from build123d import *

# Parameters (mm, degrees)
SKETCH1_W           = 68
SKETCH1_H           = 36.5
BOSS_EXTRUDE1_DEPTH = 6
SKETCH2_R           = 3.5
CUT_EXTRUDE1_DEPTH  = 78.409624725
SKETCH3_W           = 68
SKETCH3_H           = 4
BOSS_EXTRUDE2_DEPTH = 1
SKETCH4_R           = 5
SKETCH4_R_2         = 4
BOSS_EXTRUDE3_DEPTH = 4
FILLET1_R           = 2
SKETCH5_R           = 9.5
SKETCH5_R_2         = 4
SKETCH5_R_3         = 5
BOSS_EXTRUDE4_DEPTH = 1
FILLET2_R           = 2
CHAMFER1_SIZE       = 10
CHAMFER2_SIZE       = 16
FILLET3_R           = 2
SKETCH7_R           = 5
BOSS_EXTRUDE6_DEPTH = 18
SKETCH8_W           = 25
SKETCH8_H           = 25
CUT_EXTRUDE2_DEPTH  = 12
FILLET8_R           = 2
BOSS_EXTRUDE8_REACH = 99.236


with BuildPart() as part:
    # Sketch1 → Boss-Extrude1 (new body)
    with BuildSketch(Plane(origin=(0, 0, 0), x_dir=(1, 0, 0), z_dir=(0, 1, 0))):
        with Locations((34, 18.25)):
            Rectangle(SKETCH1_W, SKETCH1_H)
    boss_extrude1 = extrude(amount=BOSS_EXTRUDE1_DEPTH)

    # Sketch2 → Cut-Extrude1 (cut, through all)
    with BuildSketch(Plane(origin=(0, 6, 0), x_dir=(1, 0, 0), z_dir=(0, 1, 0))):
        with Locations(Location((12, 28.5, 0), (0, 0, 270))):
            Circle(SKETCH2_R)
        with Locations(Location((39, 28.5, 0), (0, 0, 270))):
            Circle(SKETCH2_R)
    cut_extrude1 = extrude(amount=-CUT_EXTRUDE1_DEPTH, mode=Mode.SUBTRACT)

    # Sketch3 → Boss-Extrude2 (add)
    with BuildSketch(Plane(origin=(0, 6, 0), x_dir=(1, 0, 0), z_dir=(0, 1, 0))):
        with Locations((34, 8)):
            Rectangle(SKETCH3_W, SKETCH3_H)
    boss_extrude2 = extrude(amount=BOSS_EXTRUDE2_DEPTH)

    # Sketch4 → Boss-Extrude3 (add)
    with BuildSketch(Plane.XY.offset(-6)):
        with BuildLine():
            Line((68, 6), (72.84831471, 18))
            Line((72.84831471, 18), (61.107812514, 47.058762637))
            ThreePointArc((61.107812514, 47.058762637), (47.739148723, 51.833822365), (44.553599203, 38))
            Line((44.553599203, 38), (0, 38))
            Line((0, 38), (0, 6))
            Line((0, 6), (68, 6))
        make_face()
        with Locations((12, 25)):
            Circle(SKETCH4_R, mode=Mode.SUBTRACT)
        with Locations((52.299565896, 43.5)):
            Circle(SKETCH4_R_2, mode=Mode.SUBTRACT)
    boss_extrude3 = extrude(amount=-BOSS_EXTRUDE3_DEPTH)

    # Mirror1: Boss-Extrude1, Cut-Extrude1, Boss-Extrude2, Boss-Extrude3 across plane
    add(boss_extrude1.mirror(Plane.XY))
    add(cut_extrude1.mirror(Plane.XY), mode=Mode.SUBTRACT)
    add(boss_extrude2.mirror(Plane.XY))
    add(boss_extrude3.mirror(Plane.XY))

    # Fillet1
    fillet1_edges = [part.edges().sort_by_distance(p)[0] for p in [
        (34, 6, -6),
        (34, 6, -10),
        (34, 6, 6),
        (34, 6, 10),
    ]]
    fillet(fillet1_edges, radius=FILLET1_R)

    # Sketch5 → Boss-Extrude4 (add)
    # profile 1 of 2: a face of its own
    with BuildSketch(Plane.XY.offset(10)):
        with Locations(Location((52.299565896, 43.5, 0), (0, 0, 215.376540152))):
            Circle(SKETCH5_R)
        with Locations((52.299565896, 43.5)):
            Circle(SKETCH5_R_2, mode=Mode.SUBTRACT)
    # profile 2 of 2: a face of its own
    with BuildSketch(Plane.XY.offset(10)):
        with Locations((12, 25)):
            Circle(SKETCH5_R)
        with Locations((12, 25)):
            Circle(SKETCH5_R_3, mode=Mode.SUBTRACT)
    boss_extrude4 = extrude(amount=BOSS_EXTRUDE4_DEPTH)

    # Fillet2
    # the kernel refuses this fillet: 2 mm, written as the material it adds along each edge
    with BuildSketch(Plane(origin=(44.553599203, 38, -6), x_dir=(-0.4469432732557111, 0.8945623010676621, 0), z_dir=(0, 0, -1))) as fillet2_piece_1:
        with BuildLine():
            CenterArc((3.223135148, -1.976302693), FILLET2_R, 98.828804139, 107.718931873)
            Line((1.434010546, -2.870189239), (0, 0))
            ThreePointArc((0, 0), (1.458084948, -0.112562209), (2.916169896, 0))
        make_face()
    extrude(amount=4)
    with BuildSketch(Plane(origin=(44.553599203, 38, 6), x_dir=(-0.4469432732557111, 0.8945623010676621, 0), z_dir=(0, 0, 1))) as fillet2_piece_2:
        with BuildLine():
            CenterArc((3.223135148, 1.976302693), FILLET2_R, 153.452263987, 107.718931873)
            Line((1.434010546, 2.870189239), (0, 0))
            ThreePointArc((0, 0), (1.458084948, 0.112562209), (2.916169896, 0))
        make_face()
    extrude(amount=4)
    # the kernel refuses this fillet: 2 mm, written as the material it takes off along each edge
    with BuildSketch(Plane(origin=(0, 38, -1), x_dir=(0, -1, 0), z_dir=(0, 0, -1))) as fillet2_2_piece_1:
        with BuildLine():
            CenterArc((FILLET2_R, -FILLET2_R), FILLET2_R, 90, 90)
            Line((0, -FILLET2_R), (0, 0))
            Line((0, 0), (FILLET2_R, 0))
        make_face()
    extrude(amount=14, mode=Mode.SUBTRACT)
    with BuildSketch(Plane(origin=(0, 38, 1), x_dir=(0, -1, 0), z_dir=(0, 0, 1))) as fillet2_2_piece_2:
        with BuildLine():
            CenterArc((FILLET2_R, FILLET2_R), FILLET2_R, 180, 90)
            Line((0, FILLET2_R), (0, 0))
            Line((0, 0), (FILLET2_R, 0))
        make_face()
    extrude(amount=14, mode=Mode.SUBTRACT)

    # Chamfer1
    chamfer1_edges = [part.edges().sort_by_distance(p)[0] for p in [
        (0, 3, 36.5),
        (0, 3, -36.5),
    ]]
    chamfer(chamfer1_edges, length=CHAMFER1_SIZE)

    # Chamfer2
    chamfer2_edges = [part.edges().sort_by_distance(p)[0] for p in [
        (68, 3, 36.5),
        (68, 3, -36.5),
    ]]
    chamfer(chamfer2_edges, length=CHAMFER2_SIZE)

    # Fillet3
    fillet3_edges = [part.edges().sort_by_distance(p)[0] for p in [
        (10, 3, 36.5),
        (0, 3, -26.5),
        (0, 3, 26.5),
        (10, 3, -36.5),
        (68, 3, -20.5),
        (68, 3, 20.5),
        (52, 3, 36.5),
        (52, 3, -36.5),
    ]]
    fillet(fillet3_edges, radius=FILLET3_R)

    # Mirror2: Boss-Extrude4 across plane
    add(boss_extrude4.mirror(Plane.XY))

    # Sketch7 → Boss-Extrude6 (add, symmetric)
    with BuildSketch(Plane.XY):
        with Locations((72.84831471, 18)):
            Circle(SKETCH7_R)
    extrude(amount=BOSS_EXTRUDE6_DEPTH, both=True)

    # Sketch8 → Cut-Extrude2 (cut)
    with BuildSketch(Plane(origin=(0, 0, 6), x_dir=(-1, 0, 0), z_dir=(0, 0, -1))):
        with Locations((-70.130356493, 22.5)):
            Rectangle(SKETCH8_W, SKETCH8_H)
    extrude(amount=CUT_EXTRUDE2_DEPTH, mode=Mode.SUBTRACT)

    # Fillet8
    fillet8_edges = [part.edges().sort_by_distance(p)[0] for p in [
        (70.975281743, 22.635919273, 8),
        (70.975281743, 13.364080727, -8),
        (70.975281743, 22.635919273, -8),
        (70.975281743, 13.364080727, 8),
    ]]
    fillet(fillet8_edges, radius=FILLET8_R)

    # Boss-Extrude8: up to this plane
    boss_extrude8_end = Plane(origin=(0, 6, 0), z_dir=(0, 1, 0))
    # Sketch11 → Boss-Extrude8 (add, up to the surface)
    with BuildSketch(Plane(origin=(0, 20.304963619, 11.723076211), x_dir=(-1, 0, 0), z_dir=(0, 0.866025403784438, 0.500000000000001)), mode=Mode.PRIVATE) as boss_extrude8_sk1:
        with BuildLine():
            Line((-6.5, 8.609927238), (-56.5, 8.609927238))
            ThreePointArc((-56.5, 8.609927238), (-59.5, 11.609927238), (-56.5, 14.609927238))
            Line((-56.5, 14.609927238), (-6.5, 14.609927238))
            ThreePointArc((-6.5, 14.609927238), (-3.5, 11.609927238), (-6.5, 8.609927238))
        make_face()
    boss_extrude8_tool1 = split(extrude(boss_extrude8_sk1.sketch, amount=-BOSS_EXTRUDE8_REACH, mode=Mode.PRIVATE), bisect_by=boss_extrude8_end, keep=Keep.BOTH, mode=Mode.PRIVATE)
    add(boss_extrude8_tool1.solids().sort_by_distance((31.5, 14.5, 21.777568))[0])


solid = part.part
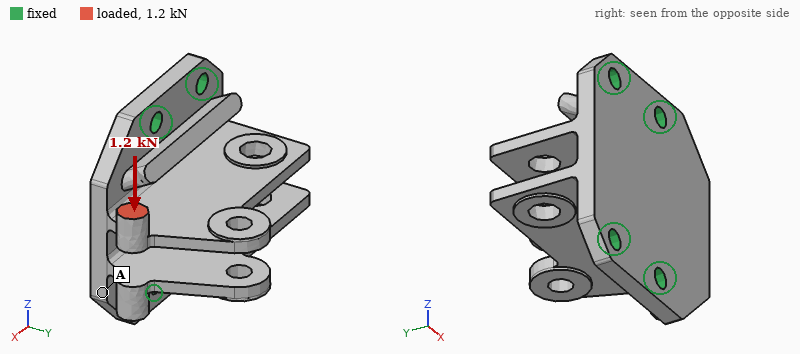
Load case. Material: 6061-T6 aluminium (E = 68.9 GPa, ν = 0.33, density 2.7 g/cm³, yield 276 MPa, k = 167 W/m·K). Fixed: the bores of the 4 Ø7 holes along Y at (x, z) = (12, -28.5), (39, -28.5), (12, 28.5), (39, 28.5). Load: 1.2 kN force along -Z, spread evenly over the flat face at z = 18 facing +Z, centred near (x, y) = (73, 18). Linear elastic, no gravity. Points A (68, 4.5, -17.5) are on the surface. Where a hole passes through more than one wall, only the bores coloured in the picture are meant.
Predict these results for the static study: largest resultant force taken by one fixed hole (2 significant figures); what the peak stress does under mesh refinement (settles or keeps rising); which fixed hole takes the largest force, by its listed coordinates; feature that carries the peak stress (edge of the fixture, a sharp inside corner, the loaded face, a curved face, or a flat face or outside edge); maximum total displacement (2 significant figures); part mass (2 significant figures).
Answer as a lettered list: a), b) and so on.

a) 1.1 kN
b) keeps rising
c) (39, 28.5)
d) a sharp inside corner
e) 0.43 mm
f) 140 g
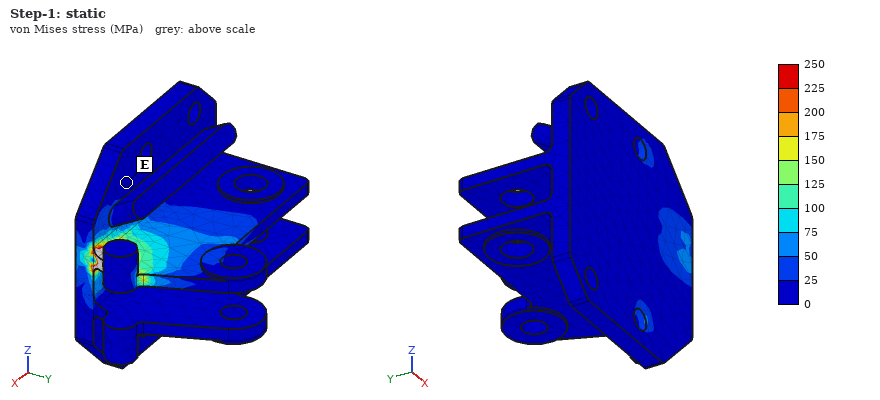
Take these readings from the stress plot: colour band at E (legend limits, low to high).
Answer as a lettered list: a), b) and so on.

a) 0 to 25 MPa
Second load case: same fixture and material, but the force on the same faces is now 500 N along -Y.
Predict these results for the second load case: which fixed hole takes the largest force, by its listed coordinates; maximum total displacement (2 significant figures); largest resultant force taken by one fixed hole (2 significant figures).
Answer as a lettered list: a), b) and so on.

a) (39, 28.5)
b) 0.16 mm
c) 770 N
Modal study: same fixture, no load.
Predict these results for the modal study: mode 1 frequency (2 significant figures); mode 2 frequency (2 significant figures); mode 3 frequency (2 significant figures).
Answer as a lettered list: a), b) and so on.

a) 2100 Hz
b) 2200 Hz
c) 3400 Hz
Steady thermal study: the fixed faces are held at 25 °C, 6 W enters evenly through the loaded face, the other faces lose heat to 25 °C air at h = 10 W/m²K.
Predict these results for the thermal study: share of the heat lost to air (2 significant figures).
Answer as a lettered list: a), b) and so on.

a) 5.3 %
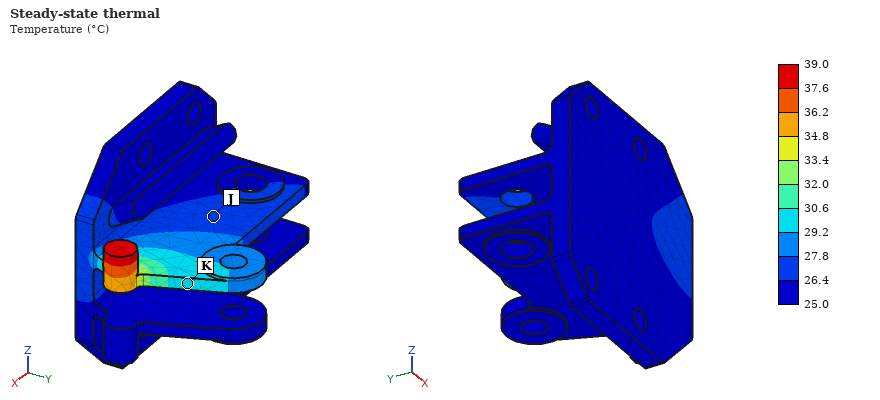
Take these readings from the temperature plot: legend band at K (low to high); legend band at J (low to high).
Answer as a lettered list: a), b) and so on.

a) 29.2 to 30.6 °C
b) 26.4 to 27.8 °C
